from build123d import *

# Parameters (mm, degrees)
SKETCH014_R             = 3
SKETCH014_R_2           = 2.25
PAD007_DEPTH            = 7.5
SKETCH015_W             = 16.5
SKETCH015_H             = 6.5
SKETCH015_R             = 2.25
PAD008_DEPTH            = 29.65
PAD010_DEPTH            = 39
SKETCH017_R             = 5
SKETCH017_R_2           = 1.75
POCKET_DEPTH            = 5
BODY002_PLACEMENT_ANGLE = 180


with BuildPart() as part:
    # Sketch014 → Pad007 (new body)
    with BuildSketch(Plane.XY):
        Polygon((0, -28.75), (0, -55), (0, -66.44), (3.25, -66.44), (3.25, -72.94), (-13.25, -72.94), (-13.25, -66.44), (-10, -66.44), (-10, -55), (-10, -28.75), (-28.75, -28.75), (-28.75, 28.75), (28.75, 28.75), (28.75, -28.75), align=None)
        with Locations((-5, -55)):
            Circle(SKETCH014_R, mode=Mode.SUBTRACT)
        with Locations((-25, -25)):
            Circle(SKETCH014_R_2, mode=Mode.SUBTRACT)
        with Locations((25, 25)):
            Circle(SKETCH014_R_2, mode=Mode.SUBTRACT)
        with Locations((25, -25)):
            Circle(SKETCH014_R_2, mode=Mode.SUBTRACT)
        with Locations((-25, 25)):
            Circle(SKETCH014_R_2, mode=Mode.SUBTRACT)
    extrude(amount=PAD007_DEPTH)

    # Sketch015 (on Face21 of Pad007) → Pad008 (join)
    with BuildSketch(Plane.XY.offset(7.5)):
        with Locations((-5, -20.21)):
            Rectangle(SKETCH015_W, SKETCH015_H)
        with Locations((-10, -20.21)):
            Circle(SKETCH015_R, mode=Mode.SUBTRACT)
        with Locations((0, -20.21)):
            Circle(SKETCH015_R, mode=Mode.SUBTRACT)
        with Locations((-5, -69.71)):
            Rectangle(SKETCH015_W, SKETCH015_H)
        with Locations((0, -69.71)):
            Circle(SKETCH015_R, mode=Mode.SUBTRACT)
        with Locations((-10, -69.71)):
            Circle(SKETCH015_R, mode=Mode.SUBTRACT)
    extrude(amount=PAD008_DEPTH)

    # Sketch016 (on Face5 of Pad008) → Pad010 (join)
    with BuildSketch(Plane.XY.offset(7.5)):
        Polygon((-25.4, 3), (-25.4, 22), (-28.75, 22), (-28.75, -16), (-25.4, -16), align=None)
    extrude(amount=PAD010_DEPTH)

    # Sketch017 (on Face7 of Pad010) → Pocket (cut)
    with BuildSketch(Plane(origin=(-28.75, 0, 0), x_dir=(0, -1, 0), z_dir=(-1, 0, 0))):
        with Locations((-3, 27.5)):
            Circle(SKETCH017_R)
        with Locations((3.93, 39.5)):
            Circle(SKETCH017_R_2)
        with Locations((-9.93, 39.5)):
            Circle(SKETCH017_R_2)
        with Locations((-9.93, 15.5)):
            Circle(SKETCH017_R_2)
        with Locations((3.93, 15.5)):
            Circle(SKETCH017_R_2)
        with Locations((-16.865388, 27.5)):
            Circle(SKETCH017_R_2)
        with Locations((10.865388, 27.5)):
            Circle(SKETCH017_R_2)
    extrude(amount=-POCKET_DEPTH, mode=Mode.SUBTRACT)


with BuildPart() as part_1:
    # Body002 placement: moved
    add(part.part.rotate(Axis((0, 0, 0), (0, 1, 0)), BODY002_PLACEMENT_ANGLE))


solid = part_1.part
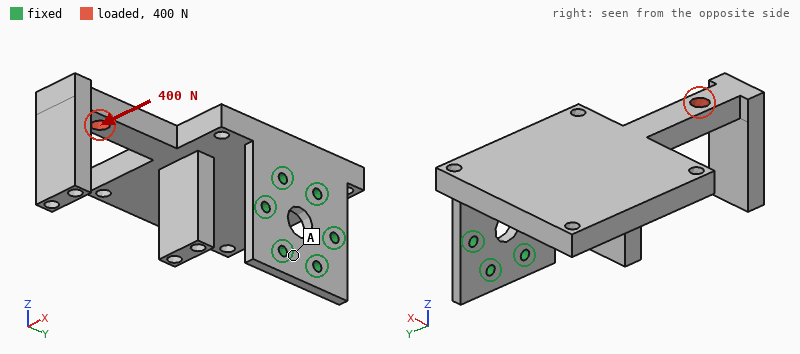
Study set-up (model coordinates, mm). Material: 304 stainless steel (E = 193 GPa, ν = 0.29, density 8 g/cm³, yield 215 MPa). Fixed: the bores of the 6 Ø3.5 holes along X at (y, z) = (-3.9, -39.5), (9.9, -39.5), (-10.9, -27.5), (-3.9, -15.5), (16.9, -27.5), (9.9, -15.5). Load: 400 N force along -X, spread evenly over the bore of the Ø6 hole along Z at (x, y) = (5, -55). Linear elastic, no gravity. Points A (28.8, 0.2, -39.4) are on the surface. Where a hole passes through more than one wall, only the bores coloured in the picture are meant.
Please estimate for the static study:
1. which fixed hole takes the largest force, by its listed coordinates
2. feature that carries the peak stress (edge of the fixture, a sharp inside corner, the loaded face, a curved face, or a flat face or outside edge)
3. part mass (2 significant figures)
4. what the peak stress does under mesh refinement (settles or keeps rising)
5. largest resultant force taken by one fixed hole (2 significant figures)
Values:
(-3.9, -15.5)
edge of the fixture
290 g
keeps rising
1.4 kN
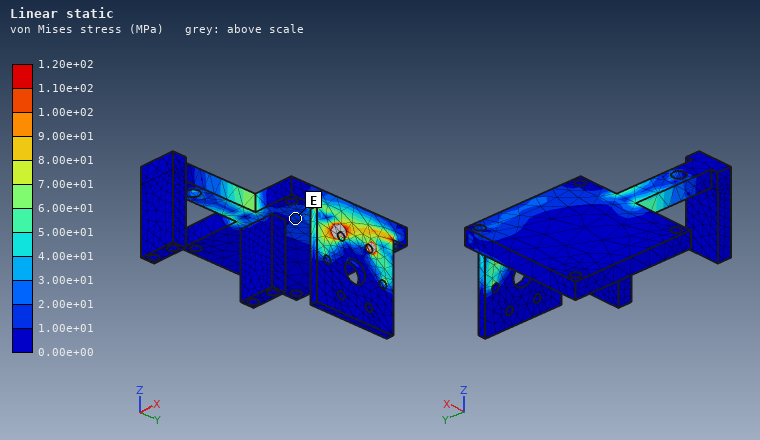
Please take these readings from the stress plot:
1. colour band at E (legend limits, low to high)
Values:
1.00e+01 to 2.00e+01 MPa
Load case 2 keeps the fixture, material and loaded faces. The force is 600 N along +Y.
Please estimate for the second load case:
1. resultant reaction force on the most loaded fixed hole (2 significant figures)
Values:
770 N
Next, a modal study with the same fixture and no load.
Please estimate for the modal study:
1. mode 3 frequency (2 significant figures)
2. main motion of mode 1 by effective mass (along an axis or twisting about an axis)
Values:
970 Hz
along Z
